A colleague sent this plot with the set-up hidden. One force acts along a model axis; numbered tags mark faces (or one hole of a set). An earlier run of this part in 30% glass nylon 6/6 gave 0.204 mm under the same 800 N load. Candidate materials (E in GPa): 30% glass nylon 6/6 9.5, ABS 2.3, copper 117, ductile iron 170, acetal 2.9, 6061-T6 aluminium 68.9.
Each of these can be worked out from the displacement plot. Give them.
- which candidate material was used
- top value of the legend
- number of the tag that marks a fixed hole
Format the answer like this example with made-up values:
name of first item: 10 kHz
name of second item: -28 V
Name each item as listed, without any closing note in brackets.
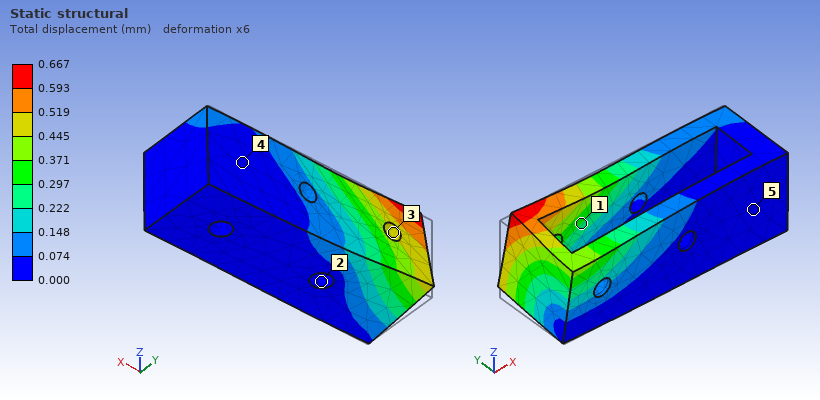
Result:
which candidate material was used: acetal
top value of the legend: 0.667 mm
number of the tag that marks a fixed hole: 2
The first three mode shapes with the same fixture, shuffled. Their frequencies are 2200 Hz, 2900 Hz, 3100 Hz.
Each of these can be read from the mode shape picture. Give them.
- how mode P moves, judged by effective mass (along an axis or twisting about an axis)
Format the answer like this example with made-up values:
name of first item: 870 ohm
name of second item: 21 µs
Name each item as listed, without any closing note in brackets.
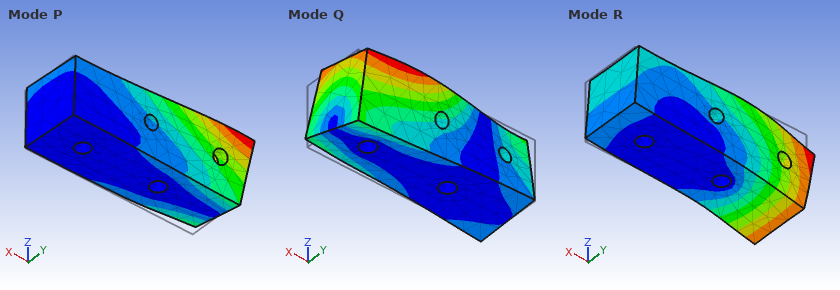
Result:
how mode P moves, judged by effective mass: along Y
